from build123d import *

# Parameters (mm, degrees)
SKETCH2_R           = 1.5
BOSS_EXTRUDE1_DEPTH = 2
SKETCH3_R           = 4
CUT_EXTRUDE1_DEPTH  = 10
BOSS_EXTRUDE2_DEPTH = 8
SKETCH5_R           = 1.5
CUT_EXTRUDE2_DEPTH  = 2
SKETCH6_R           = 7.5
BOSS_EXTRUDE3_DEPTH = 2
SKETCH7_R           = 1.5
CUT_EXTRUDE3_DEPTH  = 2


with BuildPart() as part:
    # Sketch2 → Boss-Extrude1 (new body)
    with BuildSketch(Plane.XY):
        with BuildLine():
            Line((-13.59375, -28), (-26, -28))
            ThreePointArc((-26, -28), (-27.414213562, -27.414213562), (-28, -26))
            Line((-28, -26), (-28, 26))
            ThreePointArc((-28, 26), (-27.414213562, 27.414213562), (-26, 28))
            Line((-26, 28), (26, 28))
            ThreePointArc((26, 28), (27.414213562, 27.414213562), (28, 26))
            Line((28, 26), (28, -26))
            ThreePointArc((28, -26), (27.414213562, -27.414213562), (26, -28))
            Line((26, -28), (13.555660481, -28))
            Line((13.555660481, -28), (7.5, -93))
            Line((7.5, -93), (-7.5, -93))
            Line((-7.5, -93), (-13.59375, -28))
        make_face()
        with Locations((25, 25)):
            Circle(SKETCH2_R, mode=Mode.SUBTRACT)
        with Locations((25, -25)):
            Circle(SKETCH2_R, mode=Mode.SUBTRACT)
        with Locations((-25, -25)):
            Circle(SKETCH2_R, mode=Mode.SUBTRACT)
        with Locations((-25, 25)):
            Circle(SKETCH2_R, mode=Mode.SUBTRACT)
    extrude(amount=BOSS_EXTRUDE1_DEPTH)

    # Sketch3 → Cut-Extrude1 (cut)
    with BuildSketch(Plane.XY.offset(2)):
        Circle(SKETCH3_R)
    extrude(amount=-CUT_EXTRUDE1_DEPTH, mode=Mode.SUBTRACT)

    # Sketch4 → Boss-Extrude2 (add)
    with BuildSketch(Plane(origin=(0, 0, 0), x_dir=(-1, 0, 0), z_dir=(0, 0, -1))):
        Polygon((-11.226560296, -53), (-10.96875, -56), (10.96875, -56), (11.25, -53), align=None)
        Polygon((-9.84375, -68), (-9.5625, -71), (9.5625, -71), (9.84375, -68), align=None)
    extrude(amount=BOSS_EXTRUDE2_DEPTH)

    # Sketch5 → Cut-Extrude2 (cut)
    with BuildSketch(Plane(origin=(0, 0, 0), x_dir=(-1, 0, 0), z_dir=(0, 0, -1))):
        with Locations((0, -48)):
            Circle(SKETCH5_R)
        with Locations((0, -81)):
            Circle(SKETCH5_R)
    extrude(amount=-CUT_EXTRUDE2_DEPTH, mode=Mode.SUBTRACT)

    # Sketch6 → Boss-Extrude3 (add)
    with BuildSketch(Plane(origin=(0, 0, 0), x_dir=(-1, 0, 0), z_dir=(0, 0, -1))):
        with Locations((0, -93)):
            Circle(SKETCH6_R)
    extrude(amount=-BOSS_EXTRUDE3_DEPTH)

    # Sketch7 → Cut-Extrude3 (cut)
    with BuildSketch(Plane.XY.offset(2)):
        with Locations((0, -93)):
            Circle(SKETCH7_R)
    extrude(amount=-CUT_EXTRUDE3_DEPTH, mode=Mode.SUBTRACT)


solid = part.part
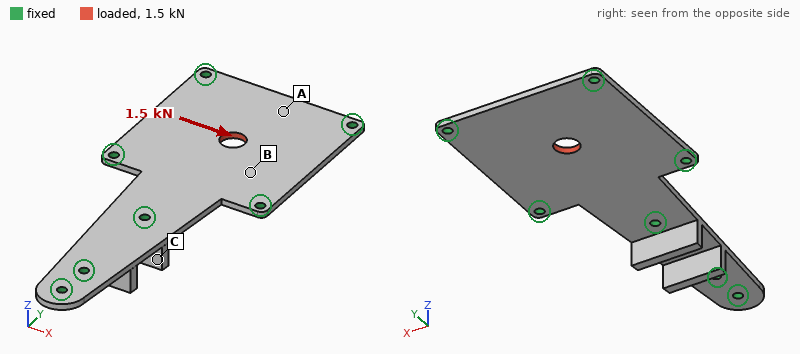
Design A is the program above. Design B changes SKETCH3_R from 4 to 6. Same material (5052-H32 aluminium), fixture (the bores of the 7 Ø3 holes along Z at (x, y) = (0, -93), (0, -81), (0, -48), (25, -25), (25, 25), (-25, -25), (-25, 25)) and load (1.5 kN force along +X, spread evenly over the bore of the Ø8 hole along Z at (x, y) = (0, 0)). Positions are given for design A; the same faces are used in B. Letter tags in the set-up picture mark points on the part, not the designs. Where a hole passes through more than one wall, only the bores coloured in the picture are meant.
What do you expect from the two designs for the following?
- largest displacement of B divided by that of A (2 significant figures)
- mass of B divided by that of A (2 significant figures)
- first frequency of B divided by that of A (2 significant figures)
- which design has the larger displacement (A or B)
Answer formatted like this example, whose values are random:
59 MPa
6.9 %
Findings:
0.90
0.99
1.0
A
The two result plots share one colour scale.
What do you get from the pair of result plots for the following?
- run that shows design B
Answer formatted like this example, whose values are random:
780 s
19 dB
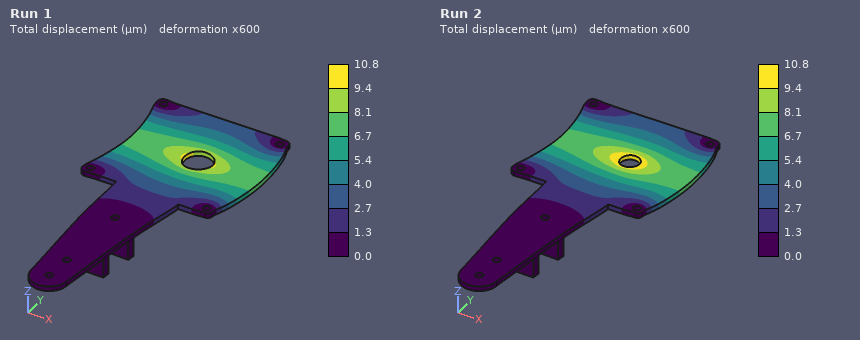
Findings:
Run 1
